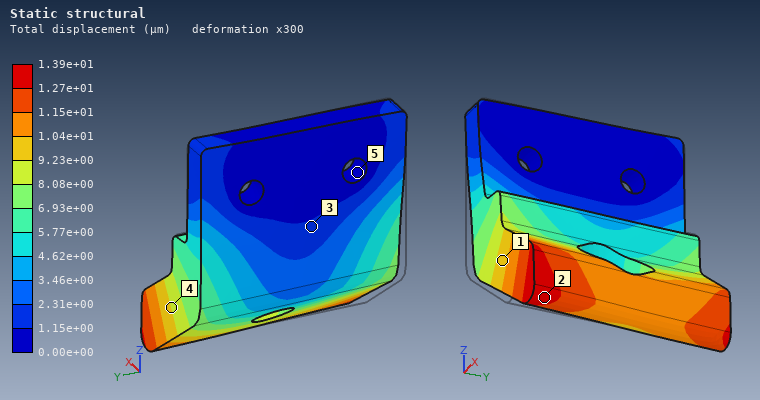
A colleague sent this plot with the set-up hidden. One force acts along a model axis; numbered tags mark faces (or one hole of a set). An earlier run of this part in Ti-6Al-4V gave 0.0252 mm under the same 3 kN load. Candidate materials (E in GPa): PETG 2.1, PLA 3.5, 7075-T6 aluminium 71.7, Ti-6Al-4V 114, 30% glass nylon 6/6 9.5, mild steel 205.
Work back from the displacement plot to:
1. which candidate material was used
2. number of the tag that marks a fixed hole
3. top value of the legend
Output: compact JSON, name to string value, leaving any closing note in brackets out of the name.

{"which candidate material was used": "mild steel", "number of the tag that marks a fixed hole": "5", "top value of the legend": "1.39e+01 µm"}
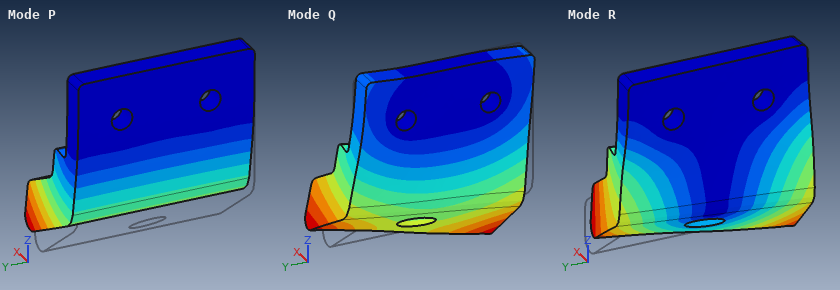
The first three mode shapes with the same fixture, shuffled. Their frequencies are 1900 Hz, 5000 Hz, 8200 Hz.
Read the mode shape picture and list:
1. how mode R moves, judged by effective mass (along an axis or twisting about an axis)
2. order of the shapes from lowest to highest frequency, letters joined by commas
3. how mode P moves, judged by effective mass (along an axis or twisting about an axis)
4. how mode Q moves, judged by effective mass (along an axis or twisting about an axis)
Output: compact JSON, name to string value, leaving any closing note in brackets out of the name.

{"how mode R moves, judged by effective mass": "along Y", "order of the shapes from lowest to highest frequency, letters joined by commas": "P, R, Q", "how mode P moves, judged by effective mass": "along X", "how mode Q moves, judged by effective mass": "along Y"}
